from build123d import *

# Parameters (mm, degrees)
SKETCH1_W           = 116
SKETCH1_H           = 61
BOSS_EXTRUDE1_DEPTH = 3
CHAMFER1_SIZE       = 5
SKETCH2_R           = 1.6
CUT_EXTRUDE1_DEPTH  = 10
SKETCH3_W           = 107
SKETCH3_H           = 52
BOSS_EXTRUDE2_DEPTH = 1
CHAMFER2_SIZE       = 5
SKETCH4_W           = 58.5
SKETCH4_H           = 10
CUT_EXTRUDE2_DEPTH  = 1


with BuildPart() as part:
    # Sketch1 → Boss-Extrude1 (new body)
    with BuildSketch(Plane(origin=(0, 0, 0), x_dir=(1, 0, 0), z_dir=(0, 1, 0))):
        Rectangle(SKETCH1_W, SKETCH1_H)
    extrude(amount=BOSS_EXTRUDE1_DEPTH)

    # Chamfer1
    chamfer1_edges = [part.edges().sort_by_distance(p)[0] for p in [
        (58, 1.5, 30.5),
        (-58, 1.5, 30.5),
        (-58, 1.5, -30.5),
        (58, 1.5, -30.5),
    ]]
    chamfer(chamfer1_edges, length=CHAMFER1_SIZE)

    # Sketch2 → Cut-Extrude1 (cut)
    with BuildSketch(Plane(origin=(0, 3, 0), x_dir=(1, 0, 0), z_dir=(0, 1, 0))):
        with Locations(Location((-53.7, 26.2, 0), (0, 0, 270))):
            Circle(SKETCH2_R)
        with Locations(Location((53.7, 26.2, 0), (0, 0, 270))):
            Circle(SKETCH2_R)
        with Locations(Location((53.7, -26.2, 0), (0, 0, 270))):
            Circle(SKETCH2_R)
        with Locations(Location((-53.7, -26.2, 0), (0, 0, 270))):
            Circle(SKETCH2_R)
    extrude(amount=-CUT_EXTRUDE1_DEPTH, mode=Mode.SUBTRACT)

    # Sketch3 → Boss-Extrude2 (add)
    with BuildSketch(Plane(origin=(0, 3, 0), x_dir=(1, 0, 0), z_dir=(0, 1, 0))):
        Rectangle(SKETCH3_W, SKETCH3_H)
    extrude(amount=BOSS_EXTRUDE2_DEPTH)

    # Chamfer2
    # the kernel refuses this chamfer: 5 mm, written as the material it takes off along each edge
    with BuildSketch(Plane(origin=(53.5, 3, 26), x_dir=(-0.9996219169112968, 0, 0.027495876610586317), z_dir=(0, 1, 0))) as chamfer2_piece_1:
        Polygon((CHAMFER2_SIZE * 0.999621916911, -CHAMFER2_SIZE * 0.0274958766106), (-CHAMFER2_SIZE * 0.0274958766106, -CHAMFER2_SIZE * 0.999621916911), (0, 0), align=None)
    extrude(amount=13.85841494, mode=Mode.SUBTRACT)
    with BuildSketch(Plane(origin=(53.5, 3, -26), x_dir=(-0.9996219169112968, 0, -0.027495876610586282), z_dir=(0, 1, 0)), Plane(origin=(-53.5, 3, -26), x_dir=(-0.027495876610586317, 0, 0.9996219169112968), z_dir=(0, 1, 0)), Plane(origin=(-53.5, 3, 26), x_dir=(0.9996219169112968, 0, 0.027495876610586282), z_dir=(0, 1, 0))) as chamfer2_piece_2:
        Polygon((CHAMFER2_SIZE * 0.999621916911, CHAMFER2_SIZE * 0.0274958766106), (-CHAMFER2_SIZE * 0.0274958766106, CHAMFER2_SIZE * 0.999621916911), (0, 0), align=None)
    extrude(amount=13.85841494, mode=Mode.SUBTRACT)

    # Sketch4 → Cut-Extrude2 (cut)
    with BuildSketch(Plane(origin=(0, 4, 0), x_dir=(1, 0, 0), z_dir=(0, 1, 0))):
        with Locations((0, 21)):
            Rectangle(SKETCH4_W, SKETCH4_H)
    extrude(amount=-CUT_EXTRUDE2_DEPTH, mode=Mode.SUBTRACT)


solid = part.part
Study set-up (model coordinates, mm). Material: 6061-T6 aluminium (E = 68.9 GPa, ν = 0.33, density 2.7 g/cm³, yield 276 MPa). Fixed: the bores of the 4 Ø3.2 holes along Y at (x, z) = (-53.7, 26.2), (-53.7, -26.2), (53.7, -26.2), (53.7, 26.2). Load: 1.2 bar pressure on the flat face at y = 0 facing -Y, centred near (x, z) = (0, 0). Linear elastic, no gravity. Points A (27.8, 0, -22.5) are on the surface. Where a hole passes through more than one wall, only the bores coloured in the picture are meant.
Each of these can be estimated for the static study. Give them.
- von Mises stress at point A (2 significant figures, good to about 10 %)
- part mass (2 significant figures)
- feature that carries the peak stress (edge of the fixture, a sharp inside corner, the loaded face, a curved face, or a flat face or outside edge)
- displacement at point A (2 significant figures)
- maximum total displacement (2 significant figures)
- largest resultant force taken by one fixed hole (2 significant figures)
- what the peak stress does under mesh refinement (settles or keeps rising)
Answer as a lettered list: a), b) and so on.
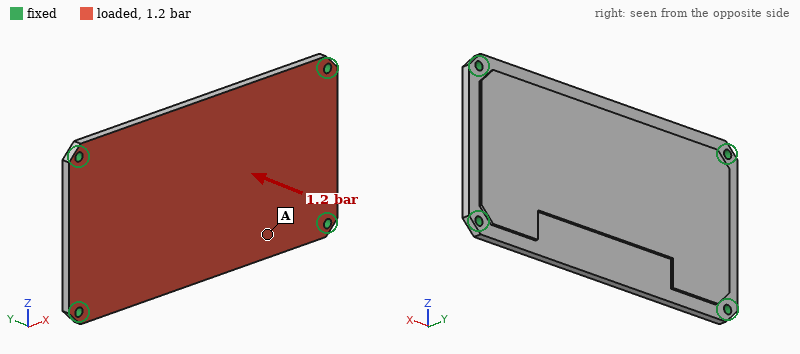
a) 18 MPa
b) 70 g
c) edge of the fixture
d) 0.15 mm
e) 0.27 mm
f) 310 N
g) keeps rising
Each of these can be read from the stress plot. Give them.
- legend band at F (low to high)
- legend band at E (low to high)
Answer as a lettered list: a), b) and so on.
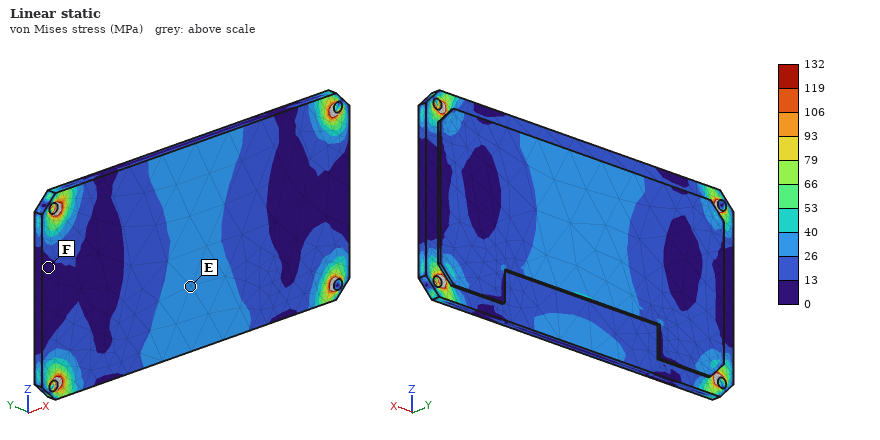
a) 0 to 13 MPa
b) 26 to 40 MPa
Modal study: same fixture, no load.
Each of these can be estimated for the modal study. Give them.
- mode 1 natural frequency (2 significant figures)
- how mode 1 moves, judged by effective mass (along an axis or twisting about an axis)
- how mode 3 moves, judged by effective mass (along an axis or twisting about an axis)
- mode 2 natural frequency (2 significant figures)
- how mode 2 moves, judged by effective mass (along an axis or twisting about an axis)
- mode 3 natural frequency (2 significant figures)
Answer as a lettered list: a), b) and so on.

a) 1300 Hz
b) along Y
c) twisting about Z
d) 2500 Hz
e) twisting about X
f) 3600 Hz
